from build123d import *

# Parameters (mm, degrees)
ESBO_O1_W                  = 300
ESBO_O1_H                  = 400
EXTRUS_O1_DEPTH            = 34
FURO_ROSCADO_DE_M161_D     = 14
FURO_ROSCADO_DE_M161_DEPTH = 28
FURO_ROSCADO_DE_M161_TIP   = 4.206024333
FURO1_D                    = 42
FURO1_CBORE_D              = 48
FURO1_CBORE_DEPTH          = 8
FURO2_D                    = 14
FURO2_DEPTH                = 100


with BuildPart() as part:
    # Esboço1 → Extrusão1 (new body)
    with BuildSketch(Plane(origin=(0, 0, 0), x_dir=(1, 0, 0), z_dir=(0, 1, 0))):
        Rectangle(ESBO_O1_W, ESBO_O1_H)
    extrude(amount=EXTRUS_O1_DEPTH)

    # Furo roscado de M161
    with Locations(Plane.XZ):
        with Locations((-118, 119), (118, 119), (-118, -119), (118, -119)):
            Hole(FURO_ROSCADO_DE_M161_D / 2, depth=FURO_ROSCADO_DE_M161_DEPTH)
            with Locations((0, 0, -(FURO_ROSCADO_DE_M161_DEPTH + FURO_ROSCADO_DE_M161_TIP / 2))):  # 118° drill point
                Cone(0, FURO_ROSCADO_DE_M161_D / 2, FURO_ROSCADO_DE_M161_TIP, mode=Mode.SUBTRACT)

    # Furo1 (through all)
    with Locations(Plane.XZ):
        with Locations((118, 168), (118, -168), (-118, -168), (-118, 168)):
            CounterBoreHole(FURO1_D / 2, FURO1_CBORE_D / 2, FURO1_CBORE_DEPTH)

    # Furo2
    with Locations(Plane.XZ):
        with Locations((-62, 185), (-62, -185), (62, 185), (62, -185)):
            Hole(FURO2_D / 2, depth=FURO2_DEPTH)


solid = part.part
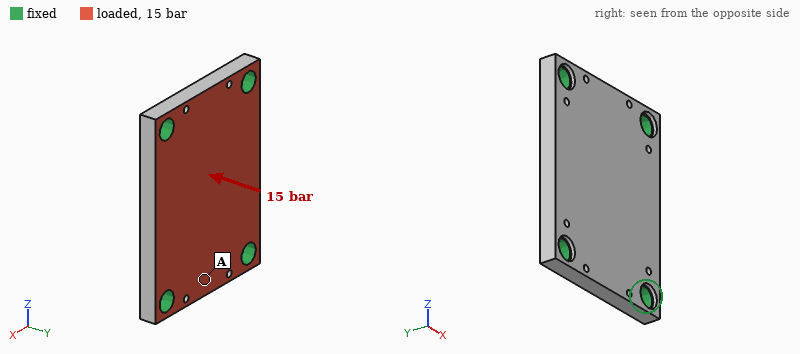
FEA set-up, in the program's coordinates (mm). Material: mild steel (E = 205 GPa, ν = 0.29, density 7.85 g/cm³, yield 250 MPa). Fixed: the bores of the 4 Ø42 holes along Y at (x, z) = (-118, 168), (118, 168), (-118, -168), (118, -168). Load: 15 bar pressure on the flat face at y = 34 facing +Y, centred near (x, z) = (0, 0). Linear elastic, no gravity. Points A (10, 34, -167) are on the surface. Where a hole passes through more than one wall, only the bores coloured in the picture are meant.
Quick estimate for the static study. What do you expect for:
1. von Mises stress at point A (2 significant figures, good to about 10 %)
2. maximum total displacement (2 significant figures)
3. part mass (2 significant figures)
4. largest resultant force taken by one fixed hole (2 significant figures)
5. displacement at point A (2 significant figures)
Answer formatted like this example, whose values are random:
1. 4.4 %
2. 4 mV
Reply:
1. 21 MPa
2. 0.11 mm
3. 30 kg
4. 44 kN
5. 0.027 mm
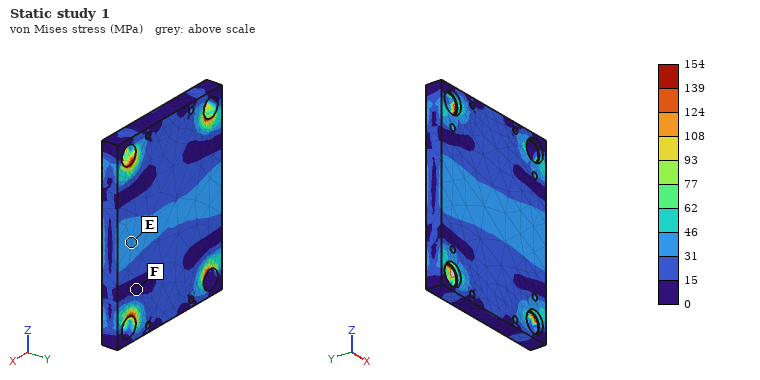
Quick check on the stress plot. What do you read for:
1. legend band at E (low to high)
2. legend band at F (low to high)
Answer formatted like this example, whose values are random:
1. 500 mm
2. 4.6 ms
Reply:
1. 31 to 46 MPa
2. 0 to 15 MPa
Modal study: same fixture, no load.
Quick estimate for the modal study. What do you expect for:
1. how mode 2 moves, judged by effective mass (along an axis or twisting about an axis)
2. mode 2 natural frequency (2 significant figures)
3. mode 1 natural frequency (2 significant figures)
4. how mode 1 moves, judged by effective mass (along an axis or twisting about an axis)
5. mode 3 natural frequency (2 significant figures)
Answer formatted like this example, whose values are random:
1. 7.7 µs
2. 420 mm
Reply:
1. twisting about Z
2. 1900 Hz
3. 1300 Hz
4. along Y
5. 2800 Hz
